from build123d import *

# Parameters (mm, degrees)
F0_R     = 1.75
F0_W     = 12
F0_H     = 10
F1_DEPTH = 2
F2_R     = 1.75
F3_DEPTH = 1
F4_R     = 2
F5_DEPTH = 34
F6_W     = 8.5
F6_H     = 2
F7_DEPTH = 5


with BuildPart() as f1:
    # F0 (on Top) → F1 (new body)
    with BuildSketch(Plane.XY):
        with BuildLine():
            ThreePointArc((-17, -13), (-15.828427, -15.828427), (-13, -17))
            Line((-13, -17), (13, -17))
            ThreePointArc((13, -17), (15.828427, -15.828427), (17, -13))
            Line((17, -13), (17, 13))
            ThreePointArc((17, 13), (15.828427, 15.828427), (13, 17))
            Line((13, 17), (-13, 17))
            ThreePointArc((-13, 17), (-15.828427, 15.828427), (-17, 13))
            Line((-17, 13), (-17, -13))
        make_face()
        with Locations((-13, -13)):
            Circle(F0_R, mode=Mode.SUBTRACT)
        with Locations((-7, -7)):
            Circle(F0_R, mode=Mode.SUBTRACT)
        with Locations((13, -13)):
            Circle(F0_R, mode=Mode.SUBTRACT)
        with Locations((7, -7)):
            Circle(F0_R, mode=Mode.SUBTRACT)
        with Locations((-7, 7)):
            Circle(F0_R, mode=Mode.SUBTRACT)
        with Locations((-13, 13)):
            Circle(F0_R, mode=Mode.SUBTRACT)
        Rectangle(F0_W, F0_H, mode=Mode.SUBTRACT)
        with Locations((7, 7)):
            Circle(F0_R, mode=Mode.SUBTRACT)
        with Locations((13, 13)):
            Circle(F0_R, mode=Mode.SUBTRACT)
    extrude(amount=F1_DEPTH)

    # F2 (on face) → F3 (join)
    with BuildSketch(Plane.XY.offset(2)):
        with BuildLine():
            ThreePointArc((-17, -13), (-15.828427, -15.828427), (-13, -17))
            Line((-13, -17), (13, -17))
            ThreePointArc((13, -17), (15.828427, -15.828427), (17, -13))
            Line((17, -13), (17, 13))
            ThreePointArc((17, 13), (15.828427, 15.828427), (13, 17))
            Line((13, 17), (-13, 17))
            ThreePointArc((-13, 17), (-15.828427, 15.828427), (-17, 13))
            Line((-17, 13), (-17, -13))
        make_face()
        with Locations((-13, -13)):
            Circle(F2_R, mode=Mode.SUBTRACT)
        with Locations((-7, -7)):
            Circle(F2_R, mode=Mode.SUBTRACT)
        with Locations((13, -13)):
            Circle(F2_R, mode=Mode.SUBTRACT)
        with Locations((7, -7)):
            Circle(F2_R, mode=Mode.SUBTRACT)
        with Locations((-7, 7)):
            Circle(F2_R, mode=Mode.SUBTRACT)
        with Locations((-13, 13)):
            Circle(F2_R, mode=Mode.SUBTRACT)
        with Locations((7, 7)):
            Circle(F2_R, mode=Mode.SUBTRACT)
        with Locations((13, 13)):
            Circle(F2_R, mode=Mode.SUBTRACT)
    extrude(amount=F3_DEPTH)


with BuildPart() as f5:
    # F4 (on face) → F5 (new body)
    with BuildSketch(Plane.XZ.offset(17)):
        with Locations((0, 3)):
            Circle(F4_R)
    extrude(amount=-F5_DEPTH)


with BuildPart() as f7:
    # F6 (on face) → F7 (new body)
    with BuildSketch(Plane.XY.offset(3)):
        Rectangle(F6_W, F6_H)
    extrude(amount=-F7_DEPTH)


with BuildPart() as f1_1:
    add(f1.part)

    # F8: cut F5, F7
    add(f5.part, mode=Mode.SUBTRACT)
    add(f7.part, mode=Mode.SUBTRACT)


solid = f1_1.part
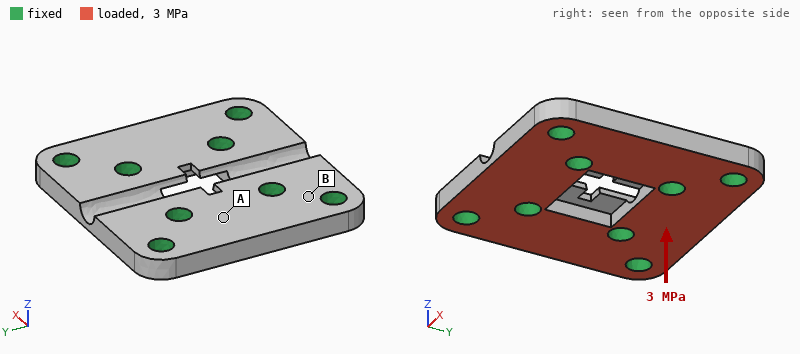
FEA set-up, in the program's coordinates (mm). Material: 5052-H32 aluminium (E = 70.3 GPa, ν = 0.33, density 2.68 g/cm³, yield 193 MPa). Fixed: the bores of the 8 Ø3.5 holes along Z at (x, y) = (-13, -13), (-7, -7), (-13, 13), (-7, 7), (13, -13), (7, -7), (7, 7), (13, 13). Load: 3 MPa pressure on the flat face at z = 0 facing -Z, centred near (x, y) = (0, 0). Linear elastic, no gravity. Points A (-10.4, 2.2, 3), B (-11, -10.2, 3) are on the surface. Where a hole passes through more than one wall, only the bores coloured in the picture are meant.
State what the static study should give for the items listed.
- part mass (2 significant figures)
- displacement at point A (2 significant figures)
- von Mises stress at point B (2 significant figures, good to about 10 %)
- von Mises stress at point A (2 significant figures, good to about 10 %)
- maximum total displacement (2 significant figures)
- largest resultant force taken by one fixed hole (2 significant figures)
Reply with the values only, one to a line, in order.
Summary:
7.4 g
4.0 µm
28 MPa
15 MPa
15 µm
420 N
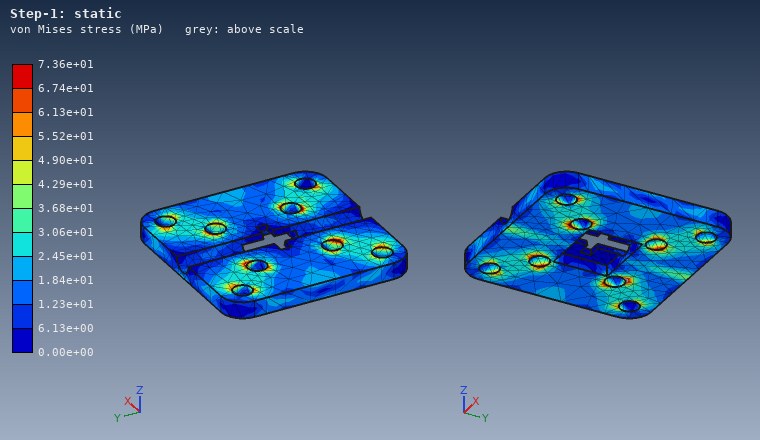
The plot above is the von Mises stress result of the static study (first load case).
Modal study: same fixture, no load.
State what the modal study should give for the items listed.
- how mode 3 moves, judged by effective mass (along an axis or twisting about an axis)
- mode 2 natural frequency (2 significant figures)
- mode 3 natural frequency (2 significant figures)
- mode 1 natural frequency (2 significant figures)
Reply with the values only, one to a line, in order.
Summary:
twisting about X
37 kHz
39 kHz
37 kHz
